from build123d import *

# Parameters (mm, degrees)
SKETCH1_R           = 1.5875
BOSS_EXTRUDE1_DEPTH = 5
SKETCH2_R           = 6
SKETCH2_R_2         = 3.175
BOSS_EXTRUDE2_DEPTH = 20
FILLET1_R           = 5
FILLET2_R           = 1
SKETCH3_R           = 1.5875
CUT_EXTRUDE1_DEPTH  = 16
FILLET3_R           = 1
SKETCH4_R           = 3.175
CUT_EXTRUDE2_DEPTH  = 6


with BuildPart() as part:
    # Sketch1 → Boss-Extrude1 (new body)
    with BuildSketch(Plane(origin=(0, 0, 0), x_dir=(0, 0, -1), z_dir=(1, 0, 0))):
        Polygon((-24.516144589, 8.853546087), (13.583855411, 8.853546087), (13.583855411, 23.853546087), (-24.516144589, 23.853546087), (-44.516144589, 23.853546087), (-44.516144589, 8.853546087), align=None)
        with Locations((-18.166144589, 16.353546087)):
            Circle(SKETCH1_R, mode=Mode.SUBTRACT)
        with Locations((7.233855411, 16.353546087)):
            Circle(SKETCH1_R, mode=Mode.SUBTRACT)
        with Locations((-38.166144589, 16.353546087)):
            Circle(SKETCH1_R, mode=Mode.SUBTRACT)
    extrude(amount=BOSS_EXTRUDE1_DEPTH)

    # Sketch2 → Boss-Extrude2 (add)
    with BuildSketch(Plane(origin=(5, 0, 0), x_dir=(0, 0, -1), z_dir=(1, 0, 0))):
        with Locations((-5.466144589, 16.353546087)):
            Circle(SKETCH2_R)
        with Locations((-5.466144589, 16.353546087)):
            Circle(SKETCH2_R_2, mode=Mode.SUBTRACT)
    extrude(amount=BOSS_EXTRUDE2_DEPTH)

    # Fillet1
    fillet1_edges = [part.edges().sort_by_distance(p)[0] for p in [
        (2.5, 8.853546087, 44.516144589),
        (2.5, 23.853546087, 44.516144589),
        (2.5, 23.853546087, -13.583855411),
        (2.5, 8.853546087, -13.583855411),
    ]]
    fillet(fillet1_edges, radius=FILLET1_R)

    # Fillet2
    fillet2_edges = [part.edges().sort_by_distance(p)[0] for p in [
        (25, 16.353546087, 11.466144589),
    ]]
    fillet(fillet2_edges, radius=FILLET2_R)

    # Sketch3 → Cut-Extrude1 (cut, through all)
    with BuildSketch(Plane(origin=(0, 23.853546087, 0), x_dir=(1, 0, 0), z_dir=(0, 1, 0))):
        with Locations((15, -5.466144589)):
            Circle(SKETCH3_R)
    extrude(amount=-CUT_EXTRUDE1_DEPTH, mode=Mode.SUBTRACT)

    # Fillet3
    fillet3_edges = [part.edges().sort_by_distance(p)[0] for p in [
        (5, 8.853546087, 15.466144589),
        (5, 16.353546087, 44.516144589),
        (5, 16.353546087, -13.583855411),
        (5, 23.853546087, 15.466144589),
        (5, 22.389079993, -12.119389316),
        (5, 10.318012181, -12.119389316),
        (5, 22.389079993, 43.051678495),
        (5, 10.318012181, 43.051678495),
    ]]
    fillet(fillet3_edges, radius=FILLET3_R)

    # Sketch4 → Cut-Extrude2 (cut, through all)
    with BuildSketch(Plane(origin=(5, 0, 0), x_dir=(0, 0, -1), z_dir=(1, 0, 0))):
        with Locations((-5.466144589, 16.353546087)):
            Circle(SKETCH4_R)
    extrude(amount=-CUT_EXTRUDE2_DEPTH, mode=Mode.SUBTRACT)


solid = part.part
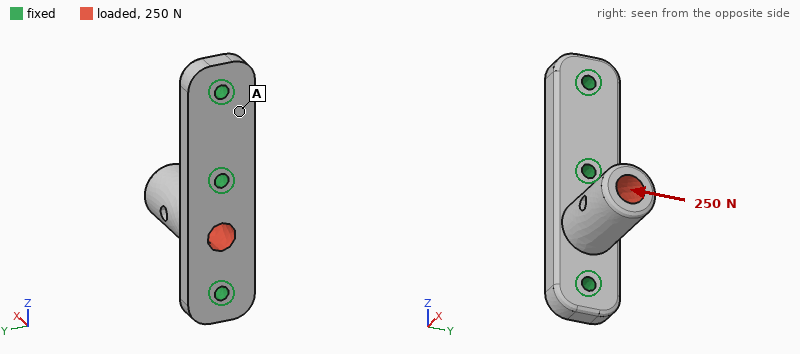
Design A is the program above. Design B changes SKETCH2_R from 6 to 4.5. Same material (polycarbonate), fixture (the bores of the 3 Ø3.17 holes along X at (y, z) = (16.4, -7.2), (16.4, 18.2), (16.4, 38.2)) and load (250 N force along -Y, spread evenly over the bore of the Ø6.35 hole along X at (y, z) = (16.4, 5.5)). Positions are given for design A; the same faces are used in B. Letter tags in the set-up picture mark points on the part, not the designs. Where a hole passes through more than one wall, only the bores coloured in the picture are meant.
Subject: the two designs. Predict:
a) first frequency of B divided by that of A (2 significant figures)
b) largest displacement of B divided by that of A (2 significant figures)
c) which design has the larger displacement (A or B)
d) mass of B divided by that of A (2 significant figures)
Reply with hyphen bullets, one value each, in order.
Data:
- 1.2
- 1.8
- B
- 0.83
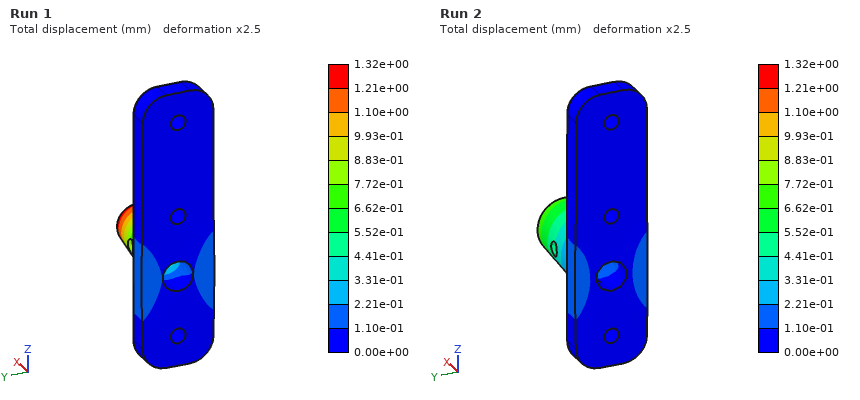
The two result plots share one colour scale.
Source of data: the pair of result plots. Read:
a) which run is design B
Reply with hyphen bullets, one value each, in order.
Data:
- Run 1
